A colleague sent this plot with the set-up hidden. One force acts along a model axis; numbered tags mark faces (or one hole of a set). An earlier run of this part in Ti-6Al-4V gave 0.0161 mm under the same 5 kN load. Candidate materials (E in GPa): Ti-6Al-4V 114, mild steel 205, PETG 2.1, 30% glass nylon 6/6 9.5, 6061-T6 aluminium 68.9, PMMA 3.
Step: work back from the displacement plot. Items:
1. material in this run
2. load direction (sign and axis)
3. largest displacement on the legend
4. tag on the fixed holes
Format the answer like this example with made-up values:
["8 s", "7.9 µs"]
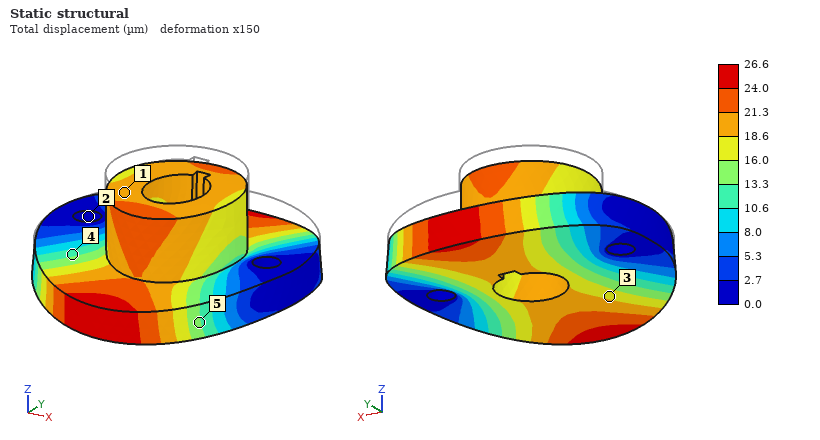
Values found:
["6061-T6 aluminium", "-Z", "26.6 µm", "2"]
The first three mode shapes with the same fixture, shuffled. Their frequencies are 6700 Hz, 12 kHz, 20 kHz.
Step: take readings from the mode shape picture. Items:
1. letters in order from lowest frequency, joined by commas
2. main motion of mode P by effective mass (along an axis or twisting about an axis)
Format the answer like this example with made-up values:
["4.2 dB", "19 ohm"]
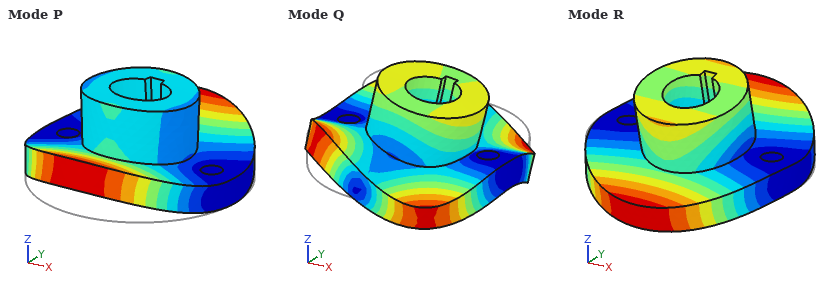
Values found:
["R, P, Q", "along Z"]
